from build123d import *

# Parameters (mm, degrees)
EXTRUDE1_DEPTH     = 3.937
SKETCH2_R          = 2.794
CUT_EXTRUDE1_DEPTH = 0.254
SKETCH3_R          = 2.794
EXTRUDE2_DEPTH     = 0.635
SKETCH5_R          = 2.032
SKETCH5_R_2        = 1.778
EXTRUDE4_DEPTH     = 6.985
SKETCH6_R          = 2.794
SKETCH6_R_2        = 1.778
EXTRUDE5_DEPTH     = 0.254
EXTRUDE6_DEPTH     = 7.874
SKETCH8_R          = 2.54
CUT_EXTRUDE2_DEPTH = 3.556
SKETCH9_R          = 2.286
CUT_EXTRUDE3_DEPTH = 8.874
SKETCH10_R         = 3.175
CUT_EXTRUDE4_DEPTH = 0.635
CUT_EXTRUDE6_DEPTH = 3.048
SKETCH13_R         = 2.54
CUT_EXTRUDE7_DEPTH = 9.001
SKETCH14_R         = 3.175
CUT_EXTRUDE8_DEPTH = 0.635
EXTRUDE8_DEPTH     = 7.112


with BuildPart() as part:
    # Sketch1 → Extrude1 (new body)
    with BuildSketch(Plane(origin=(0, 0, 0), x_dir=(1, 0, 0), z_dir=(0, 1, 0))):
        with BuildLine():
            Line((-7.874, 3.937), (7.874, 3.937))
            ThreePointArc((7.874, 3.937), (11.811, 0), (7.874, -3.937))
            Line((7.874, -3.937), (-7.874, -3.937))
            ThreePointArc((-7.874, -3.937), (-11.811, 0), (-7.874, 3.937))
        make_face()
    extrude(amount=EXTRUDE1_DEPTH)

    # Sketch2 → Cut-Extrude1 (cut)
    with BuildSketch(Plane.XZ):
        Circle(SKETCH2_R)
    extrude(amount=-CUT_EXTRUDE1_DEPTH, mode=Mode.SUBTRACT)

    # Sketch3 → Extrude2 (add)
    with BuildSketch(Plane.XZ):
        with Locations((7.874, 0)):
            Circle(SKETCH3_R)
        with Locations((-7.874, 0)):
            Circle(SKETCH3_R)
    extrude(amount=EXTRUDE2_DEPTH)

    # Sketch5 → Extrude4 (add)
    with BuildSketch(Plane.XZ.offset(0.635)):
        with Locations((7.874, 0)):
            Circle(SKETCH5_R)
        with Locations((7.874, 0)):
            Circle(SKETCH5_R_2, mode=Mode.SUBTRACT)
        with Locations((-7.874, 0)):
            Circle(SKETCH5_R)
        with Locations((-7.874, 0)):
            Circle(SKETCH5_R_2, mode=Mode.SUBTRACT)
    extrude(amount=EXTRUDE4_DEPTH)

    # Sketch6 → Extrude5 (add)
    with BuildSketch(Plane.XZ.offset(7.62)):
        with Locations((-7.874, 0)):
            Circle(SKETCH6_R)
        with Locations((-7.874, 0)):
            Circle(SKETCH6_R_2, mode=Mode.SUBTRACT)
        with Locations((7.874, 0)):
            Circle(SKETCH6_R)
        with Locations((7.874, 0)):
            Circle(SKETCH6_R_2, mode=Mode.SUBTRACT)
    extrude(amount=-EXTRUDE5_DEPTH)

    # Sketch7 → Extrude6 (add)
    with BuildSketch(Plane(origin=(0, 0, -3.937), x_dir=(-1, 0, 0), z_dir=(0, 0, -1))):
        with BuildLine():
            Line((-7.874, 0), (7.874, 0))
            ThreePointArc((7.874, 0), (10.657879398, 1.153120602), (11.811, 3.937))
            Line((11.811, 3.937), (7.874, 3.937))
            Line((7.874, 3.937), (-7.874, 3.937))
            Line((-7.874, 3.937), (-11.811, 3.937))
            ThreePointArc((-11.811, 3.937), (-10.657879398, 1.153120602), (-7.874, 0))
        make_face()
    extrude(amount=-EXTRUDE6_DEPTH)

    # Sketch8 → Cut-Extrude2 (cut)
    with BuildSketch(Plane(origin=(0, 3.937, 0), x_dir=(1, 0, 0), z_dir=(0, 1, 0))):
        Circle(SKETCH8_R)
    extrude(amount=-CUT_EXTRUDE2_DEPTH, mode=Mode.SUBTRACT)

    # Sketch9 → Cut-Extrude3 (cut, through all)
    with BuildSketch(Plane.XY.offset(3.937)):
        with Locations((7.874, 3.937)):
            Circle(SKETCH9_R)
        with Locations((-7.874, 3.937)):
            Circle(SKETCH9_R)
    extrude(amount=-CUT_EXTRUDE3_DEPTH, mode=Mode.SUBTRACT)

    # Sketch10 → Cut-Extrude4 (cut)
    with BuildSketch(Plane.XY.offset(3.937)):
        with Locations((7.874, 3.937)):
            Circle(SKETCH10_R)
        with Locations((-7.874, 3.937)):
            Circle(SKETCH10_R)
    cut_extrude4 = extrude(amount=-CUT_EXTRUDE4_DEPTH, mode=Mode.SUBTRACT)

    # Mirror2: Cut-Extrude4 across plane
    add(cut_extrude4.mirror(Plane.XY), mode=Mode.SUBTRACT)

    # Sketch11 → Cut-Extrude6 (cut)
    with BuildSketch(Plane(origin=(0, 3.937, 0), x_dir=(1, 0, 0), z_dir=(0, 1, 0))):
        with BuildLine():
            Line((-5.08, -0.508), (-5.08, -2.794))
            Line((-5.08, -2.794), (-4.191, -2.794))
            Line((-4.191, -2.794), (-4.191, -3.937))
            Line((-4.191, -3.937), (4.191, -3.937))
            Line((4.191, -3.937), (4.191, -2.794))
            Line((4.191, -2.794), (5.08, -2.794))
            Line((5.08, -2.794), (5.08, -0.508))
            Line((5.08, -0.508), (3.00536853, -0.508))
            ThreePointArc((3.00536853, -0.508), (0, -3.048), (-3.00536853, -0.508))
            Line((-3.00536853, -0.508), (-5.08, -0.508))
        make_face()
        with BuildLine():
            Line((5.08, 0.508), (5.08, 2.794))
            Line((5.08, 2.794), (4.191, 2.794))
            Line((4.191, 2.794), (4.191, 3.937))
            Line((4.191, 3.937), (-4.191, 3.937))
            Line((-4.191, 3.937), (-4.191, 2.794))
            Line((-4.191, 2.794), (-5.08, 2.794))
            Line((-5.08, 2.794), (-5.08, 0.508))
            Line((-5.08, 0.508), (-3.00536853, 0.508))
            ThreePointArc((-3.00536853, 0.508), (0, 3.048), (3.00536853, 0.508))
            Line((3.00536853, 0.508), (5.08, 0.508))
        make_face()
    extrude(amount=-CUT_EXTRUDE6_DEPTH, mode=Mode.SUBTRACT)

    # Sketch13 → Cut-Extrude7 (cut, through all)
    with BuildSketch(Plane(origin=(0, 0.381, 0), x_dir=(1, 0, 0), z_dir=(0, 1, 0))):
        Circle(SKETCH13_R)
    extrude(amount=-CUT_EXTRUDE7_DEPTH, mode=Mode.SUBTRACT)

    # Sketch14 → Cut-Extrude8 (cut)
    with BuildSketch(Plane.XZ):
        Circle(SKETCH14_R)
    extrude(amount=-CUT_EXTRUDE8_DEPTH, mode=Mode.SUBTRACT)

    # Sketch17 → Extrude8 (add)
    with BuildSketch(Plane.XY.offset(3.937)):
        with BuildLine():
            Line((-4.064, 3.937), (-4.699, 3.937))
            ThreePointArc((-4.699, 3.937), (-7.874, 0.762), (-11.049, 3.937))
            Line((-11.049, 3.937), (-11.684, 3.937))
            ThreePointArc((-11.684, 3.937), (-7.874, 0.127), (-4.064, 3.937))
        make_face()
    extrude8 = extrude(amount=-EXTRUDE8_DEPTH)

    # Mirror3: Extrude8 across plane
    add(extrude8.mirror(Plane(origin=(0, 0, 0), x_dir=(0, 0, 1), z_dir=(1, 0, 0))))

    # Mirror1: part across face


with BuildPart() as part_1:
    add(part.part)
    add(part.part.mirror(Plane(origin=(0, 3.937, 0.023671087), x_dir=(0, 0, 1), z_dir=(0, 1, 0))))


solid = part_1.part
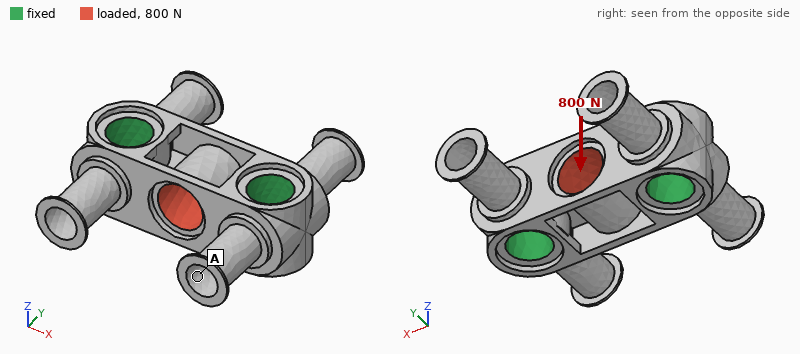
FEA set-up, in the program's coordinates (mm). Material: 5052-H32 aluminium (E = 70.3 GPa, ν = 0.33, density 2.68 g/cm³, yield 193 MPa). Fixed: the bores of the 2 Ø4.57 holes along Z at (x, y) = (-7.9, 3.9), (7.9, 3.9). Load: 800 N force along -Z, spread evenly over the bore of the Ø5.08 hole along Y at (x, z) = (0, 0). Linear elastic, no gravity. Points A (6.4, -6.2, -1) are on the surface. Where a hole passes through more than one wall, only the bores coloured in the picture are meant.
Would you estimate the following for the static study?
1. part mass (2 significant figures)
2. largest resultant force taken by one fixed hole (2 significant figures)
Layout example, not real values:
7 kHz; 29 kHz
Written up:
2.3 g; 400 N
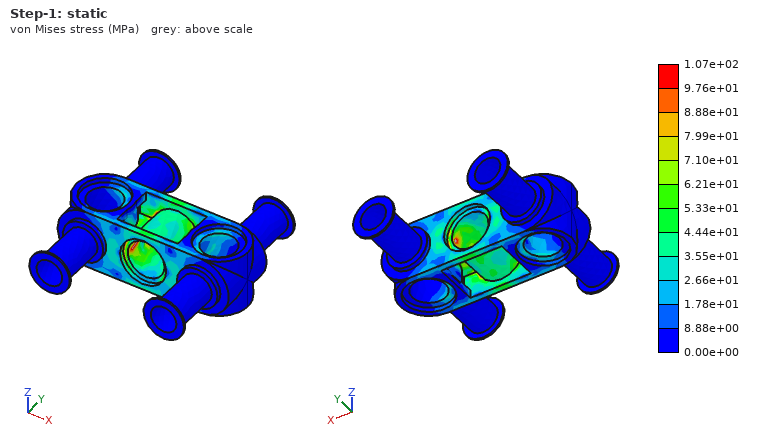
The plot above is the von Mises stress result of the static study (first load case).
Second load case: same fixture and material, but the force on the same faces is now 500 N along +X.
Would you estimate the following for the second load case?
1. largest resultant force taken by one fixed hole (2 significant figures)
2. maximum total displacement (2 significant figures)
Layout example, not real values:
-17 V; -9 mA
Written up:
250 N; 5.1 µm
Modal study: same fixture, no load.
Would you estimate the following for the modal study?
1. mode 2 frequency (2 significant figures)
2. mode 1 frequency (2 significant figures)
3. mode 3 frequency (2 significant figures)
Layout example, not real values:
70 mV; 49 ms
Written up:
43 kHz; 43 kHz; 44 kHz
